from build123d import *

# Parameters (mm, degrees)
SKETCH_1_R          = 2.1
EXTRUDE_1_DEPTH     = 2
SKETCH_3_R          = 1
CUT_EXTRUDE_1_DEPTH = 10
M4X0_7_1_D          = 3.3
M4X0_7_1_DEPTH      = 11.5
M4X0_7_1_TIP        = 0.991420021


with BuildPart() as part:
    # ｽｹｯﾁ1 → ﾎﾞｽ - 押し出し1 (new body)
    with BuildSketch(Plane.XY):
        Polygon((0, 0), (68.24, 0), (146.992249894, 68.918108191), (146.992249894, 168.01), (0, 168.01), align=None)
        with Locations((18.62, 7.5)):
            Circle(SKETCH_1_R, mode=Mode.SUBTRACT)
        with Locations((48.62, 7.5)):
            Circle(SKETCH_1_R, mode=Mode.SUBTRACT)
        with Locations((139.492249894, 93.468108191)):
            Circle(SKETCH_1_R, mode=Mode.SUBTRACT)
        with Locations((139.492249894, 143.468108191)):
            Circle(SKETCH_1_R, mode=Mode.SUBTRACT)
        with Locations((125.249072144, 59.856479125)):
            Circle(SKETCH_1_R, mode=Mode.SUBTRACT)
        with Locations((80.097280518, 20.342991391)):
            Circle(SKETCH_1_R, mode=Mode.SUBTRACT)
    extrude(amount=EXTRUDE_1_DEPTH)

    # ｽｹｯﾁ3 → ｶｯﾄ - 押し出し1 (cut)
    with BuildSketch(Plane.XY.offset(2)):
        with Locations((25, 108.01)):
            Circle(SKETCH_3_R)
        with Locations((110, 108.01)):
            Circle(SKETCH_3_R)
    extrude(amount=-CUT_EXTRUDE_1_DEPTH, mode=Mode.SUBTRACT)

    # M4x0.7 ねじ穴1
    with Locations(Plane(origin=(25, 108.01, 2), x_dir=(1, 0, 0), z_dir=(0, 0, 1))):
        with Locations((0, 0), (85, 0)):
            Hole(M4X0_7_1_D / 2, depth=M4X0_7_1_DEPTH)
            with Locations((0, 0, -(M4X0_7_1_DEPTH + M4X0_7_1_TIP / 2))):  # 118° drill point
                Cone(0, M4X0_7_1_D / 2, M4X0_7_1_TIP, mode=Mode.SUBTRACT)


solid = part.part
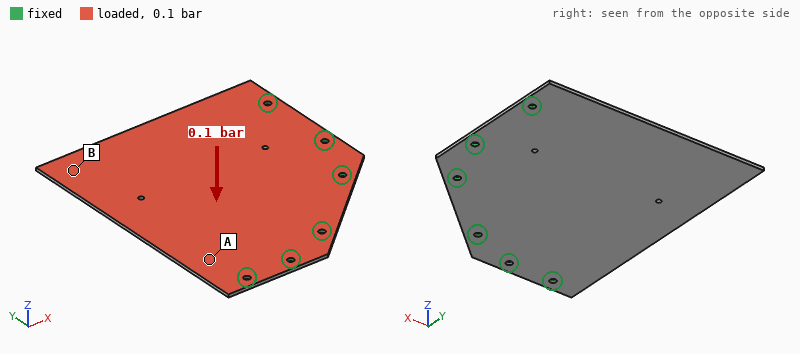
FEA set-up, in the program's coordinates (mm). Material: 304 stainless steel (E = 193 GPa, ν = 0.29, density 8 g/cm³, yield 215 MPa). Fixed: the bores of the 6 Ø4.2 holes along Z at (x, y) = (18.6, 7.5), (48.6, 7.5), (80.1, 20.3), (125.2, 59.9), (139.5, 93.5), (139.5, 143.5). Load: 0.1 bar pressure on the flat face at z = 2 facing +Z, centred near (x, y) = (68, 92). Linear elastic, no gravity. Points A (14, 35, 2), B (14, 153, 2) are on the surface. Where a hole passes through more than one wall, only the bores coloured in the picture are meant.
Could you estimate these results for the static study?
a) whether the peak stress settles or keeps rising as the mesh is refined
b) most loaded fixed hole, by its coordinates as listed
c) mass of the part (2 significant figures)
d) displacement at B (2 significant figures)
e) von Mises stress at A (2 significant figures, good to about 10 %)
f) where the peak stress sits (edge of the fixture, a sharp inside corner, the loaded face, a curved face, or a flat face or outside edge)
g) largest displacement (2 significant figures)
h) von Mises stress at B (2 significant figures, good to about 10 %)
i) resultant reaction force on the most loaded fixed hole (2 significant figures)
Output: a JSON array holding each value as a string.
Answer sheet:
["keeps rising", "(139.5, 143.5)", "350 g", "1.3 mm", "36 MPa", "edge of the fixture", "1.6 mm", "12 MPa", "79 N"]
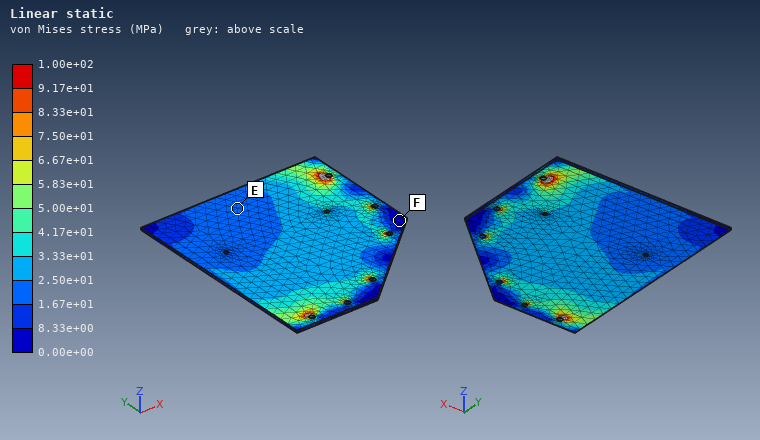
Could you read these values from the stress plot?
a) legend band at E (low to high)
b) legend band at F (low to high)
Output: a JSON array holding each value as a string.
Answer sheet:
["1.67e+01 to 2.50e+01 MPa", "0.00e+00 to 8.33e+00 MPa"]
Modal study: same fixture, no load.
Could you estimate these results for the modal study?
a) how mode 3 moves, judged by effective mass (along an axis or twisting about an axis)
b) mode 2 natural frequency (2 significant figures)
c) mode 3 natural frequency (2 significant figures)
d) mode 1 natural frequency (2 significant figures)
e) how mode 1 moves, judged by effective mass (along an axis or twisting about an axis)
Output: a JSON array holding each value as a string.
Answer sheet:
["along Z", "470 Hz", "590 Hz", "140 Hz", "along Z"]
